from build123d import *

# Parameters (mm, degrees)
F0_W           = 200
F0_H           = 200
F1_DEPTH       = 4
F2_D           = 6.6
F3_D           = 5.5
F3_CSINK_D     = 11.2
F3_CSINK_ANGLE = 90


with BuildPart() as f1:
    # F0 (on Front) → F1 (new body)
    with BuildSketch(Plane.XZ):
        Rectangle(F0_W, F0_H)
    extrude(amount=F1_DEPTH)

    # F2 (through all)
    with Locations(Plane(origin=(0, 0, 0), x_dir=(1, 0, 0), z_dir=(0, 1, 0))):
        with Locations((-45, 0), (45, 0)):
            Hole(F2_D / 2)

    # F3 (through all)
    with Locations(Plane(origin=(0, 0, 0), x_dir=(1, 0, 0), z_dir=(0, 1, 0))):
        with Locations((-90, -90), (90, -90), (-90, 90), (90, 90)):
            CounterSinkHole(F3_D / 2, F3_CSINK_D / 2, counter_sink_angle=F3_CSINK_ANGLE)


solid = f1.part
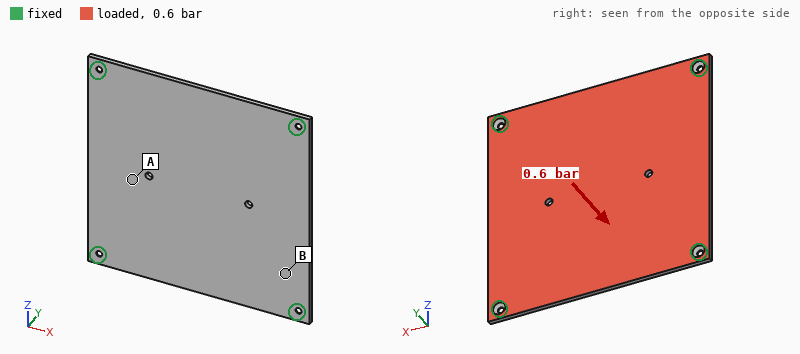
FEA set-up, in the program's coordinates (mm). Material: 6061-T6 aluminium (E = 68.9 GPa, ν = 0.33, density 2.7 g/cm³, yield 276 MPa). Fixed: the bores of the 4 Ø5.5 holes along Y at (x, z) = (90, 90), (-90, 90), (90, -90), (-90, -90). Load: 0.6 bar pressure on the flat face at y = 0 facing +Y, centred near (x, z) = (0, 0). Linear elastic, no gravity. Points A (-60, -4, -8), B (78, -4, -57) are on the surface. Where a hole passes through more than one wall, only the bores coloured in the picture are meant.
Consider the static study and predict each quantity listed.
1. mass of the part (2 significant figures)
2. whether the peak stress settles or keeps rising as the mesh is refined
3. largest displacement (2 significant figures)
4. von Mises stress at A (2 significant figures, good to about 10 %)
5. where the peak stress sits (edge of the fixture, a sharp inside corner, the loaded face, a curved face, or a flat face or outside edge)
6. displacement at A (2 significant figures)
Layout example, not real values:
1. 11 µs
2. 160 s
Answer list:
1. 430 g
2. keeps rising
3. 1.7 mm
4. 42 MPa
5. edge of the fixture
6. 1.3 mm
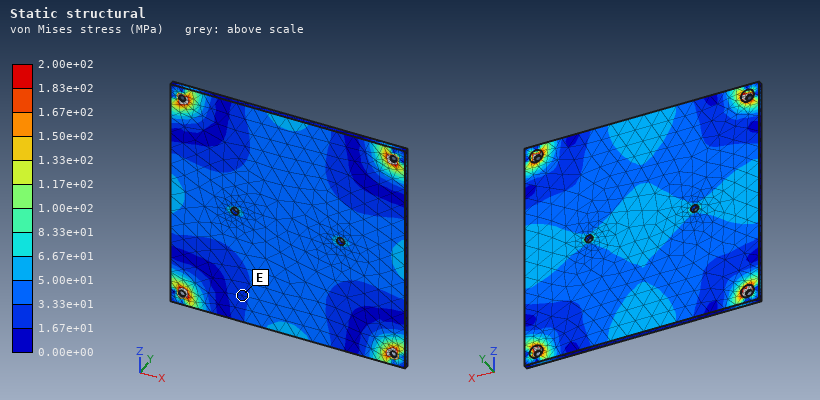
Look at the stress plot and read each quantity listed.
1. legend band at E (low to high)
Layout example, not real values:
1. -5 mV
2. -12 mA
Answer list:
1. 1.67e+01 to 3.33e+01 MPa
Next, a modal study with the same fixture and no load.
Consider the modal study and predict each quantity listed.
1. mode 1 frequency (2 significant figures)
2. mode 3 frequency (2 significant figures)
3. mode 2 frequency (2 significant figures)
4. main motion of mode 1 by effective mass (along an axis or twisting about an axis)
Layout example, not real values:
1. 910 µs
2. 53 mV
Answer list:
1. 340 Hz
2. 620 Hz
3. 620 Hz
4. along Y
